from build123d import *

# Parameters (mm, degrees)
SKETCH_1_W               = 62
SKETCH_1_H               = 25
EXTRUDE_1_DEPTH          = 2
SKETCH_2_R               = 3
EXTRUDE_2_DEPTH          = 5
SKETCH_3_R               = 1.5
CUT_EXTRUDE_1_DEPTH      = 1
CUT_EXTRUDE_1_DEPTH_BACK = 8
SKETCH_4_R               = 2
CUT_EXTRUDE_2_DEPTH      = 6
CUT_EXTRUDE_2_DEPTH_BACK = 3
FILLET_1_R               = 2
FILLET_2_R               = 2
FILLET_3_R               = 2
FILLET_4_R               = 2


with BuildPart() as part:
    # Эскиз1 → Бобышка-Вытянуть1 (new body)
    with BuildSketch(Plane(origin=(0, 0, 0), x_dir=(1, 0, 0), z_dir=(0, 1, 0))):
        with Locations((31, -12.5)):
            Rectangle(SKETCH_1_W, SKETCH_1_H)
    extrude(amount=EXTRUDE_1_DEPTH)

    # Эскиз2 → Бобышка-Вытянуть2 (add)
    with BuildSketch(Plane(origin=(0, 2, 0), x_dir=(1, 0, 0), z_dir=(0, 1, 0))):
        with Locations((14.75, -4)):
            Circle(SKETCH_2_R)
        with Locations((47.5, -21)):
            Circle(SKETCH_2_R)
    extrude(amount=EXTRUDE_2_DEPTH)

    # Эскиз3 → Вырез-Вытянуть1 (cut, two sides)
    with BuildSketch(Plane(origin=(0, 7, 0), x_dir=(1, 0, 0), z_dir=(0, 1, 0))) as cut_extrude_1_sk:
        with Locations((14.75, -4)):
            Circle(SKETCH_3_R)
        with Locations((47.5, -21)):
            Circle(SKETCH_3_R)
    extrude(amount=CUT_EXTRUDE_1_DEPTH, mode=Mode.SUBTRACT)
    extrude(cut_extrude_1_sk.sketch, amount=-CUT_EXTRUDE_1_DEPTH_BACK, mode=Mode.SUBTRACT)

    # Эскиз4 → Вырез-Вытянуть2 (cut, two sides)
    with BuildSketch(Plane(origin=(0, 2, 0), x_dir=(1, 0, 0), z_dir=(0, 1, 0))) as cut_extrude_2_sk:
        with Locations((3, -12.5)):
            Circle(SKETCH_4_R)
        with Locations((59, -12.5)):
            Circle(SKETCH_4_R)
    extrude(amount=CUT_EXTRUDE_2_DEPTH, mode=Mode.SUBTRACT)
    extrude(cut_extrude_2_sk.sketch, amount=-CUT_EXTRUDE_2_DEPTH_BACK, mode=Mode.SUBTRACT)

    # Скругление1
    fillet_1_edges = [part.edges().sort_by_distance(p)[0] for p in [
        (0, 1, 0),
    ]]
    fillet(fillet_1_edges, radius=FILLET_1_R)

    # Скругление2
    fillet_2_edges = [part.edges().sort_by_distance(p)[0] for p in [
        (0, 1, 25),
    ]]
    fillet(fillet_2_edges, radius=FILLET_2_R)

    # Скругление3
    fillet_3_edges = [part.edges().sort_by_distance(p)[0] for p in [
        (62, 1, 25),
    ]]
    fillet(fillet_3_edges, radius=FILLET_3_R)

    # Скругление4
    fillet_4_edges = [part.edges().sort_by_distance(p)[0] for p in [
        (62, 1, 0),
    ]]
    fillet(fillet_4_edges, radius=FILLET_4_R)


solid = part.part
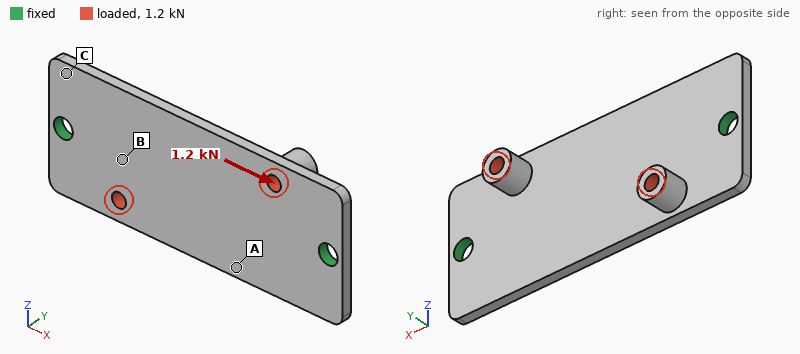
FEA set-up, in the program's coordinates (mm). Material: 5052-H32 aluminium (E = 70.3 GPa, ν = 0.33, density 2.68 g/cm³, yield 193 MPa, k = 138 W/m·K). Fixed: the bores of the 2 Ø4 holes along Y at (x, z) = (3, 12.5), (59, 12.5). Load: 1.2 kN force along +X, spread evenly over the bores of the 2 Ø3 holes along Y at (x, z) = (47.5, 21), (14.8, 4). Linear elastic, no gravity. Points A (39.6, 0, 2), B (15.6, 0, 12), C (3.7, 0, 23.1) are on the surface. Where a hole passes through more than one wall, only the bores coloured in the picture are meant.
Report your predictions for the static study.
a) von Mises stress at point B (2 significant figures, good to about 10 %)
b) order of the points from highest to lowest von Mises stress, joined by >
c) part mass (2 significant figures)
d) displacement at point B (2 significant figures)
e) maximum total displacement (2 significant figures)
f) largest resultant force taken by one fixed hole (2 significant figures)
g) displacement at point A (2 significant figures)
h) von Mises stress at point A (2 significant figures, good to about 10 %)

52 MPa
B > A > C
8.6 g
15 µm
88 µm
600 N
41 µm
30 MPa
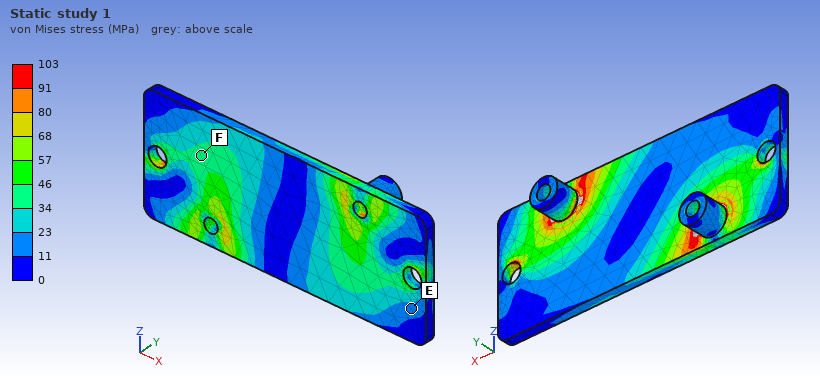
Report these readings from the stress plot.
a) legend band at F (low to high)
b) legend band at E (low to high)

34 to 46 MPa
11 to 23 MPa
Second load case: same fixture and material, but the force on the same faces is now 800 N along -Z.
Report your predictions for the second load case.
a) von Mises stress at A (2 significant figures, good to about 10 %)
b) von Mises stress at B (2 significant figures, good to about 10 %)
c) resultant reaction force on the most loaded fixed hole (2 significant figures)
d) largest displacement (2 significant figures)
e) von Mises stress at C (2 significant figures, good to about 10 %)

28 MPa
28 MPa
400 N
0.12 mm
12 MPa
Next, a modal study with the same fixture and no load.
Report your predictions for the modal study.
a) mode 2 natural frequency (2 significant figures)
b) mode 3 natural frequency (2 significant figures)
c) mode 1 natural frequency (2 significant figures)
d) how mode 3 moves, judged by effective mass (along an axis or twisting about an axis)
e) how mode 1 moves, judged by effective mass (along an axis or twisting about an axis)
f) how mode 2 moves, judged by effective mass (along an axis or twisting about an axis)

4200 Hz
8000 Hz
3200 Hz
twisting about Z
along Y
twisting about X
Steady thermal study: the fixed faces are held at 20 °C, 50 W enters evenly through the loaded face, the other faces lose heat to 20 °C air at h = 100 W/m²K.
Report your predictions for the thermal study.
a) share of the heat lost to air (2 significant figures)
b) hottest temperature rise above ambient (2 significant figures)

24 %
78 K
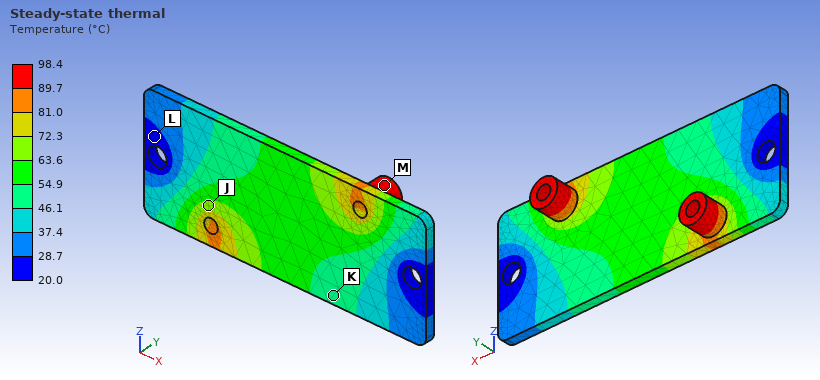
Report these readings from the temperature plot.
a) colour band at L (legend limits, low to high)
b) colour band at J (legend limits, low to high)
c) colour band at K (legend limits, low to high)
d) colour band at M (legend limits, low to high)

20.0 to 28.7 °C
63.6 to 72.3 °C
46.1 to 54.9 °C
89.7 to 98.4 °C
